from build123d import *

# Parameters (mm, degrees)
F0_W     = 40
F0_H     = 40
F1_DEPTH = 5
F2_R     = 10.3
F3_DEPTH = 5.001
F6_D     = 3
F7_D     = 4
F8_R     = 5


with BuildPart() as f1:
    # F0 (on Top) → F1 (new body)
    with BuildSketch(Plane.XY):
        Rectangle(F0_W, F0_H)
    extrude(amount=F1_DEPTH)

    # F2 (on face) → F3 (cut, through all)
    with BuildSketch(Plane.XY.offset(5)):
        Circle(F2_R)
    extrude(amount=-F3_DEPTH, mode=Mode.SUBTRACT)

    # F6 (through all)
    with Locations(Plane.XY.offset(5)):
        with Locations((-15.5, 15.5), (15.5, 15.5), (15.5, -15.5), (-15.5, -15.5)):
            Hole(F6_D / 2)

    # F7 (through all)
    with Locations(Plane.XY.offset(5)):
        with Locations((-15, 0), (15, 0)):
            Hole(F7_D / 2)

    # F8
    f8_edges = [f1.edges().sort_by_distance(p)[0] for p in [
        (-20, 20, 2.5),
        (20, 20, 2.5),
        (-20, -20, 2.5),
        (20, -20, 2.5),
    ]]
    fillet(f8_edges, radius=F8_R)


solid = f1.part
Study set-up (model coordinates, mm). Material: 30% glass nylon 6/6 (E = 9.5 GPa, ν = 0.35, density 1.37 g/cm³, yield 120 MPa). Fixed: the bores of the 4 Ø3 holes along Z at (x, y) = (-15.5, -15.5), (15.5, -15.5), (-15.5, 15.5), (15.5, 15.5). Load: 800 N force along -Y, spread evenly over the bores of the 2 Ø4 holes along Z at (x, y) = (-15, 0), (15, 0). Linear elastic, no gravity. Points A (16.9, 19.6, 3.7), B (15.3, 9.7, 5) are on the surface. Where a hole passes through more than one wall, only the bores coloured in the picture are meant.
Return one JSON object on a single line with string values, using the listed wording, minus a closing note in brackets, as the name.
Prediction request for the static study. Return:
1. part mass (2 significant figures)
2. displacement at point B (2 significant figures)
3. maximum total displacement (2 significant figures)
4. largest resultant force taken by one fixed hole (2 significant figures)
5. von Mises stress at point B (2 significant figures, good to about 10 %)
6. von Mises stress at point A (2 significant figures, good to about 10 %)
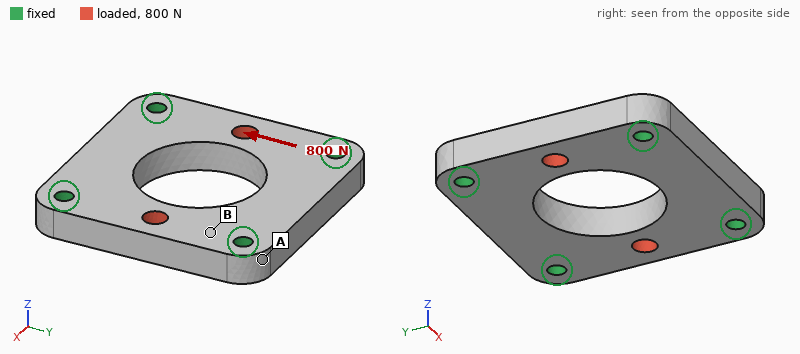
{"part mass": "8.2 g", "displacement at point B": "2.7 µm", "maximum total displacement": "7.4 µm", "largest resultant force taken by one fixed hole": "200 N", "von Mises stress at point B": "5.0 MPa", "von Mises stress at point A": "1.8 MPa"}
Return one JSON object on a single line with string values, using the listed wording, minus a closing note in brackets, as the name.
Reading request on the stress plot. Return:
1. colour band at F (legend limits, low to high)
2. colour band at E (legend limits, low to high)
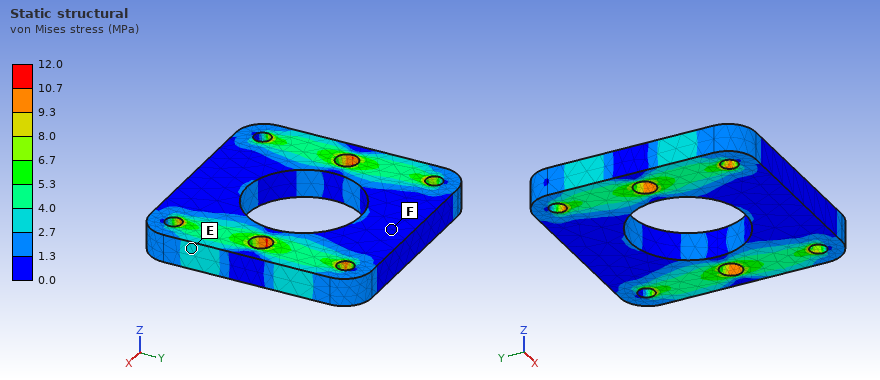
{"colour band at F": "0.0 to 1.3 MPa", "colour band at E": "2.7 to 4.0 MPa"}
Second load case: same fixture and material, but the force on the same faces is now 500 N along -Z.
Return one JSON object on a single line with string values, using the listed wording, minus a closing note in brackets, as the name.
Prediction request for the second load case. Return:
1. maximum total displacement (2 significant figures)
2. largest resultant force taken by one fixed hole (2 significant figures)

{"maximum total displacement": "54 µm", "largest resultant force taken by one fixed hole": "130 N"}
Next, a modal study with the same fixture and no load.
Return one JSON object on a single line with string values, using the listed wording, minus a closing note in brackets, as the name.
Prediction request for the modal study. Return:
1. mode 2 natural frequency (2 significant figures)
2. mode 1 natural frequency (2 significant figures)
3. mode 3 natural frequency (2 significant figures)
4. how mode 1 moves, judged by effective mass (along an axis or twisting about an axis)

{"mode 2 natural frequency": "13 kHz", "mode 1 natural frequency": "11 kHz", "mode 3 natural frequency": "13 kHz", "how mode 1 moves, judged by effective mass": "along Z"}
